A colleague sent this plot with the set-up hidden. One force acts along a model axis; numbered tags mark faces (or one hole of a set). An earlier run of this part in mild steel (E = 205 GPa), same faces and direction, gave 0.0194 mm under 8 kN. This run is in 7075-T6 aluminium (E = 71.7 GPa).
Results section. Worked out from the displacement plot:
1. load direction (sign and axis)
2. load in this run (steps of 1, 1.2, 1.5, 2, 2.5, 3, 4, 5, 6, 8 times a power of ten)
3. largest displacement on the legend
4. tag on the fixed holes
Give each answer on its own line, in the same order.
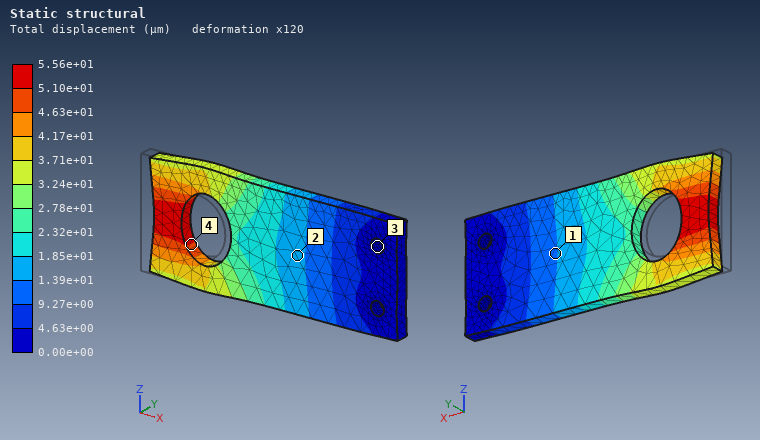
+X
8 kN
5.56e+01 µm
3
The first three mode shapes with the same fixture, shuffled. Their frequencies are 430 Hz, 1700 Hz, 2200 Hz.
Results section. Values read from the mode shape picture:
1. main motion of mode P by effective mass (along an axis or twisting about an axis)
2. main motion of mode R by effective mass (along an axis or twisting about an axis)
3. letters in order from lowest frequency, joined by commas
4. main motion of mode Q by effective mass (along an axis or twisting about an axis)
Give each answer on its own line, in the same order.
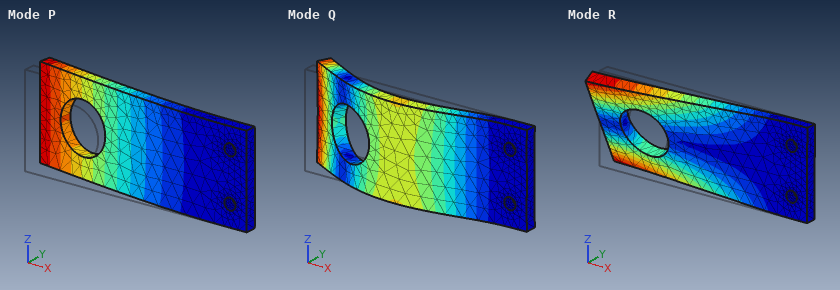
along Y
twisting about X
P, R, Q
along Y
